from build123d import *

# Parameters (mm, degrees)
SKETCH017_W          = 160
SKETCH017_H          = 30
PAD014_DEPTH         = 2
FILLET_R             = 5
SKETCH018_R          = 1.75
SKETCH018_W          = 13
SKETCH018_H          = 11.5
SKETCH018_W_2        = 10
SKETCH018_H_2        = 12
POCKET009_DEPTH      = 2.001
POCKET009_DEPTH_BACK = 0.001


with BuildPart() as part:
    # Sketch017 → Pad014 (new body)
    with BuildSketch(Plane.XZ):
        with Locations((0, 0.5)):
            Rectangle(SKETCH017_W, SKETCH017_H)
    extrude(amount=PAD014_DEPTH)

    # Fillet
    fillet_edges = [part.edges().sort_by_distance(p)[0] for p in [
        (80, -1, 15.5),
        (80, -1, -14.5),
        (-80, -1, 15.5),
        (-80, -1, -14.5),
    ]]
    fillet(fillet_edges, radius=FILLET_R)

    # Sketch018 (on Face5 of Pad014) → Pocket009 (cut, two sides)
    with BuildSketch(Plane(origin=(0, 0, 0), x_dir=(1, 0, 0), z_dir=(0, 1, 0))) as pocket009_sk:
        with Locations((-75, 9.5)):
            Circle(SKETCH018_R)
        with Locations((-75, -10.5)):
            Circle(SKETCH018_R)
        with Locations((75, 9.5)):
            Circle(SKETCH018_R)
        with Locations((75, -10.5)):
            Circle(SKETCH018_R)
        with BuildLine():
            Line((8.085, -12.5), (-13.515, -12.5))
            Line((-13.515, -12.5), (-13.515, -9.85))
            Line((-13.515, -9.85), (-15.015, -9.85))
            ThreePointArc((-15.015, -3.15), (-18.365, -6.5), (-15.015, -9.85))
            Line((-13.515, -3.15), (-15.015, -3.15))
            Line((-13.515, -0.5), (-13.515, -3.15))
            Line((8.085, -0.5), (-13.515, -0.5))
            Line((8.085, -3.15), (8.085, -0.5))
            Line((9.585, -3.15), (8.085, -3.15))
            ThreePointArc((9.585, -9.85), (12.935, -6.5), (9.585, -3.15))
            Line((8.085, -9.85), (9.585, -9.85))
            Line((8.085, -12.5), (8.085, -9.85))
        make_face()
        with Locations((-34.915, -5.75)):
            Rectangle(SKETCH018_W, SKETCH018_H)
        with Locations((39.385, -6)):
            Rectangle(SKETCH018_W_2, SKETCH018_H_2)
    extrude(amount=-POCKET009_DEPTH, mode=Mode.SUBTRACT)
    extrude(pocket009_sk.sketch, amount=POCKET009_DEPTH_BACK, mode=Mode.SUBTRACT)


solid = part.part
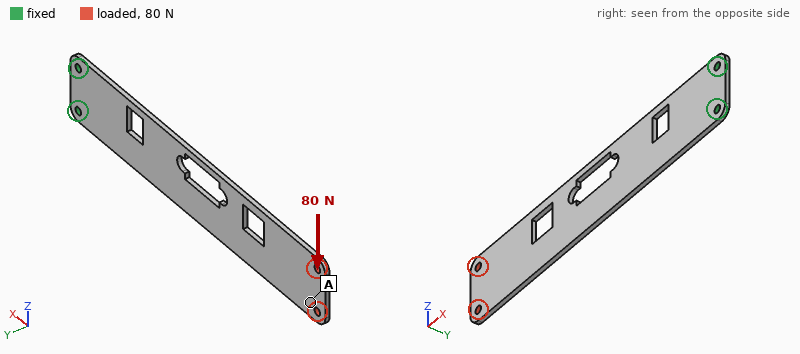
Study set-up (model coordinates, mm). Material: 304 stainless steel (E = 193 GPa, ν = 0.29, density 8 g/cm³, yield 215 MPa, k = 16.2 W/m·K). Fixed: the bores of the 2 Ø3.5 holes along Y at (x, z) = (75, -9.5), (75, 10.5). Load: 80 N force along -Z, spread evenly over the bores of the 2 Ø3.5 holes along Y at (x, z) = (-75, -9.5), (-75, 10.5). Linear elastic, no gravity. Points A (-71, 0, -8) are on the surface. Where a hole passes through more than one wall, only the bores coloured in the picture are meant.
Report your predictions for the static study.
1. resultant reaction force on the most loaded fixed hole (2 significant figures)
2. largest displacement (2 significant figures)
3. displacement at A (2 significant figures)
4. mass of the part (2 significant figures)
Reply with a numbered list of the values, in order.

1. 560 N
2. 0.15 mm
3. 0.13 mm
4. 66 g
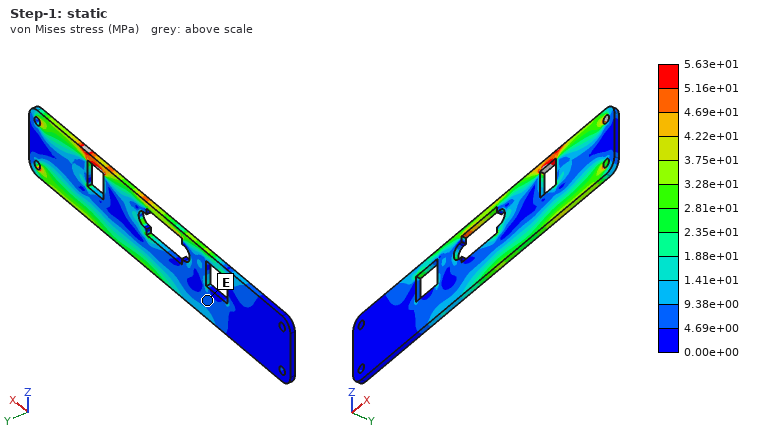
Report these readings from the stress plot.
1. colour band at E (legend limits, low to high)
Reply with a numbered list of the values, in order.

1. 4.69e+00 to 9.38e+00 MPa
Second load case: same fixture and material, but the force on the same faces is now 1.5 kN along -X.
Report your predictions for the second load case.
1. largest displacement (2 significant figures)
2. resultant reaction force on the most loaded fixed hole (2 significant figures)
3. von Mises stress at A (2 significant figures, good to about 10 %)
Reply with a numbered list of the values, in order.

1. 73 µm
2. 760 N
3. 32 MPa
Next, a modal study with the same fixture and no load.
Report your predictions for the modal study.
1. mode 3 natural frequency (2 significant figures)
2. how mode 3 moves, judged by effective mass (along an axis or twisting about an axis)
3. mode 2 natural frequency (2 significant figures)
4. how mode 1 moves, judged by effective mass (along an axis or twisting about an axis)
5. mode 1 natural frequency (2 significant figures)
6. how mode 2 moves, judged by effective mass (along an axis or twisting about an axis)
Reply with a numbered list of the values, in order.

1. 630 Hz
2. twisting about X
3. 400 Hz
4. along Y
5. 64 Hz
6. along Y
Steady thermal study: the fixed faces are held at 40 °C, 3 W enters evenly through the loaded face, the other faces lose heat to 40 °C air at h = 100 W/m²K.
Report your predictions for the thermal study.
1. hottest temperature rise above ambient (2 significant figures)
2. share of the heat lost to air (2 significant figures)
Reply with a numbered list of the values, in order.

1. 36 K
2. 100 %
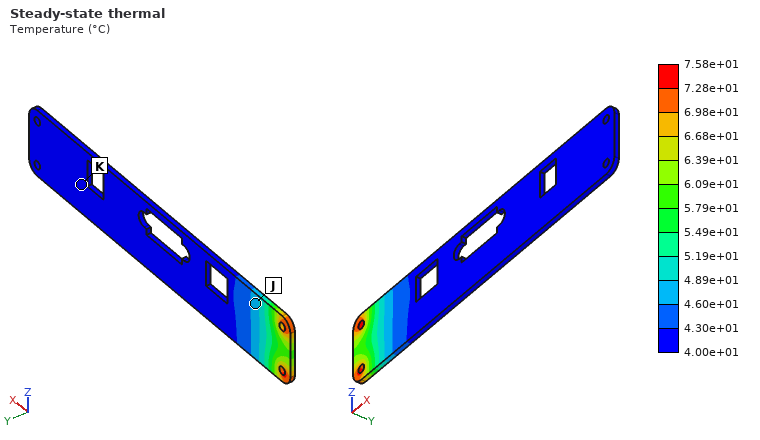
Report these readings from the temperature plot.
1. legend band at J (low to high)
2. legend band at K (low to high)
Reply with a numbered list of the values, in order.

1. 4.60e+01 to 4.89e+01 °C
2. 4.00e+01 to 4.30e+01 °C
